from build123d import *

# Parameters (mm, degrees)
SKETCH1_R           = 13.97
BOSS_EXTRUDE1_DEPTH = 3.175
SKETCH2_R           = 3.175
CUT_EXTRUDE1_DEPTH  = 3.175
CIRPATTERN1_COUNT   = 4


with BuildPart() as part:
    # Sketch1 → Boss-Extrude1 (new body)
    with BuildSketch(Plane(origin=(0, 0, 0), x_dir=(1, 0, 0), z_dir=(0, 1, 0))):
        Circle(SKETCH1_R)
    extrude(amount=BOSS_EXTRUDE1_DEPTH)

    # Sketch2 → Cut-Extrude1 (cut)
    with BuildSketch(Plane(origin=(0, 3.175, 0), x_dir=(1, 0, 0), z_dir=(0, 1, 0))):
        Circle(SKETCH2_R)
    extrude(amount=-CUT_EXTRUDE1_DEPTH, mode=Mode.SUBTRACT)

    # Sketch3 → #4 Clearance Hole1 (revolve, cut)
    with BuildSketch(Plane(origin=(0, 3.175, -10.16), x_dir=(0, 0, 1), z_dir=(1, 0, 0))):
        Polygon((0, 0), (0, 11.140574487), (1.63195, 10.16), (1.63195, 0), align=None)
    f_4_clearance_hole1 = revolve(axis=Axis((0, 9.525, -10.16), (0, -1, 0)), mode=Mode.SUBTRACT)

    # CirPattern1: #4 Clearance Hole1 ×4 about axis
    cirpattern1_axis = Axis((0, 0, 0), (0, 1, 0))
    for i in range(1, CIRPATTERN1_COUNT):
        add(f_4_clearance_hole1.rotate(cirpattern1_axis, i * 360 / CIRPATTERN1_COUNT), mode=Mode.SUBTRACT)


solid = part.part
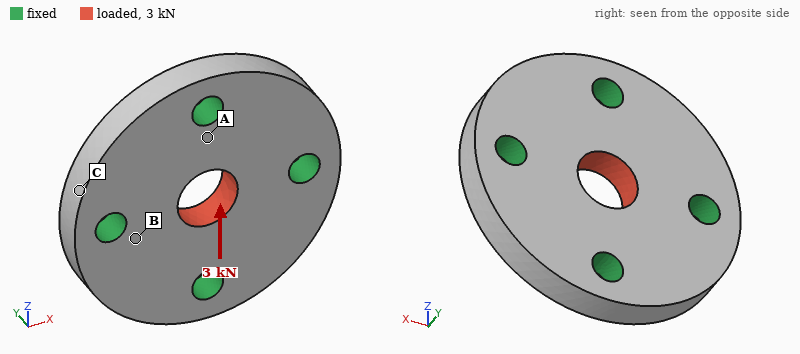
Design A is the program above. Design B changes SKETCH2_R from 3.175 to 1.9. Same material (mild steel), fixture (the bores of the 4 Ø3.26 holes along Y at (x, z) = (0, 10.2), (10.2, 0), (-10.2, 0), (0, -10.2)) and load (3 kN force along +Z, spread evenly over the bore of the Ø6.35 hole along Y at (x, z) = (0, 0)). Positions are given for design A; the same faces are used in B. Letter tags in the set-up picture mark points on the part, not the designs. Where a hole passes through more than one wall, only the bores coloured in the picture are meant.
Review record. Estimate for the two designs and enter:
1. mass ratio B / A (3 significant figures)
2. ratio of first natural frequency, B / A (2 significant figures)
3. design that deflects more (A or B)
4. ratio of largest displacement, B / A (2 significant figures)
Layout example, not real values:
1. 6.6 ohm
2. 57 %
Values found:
1. 1.04
2. 1.0
3. B
4. 1.3
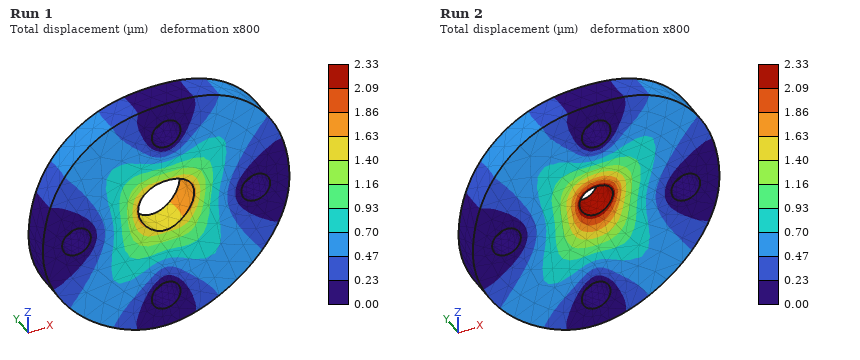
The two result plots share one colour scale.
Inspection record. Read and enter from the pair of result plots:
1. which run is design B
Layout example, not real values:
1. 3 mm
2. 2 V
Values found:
1. Run 2
